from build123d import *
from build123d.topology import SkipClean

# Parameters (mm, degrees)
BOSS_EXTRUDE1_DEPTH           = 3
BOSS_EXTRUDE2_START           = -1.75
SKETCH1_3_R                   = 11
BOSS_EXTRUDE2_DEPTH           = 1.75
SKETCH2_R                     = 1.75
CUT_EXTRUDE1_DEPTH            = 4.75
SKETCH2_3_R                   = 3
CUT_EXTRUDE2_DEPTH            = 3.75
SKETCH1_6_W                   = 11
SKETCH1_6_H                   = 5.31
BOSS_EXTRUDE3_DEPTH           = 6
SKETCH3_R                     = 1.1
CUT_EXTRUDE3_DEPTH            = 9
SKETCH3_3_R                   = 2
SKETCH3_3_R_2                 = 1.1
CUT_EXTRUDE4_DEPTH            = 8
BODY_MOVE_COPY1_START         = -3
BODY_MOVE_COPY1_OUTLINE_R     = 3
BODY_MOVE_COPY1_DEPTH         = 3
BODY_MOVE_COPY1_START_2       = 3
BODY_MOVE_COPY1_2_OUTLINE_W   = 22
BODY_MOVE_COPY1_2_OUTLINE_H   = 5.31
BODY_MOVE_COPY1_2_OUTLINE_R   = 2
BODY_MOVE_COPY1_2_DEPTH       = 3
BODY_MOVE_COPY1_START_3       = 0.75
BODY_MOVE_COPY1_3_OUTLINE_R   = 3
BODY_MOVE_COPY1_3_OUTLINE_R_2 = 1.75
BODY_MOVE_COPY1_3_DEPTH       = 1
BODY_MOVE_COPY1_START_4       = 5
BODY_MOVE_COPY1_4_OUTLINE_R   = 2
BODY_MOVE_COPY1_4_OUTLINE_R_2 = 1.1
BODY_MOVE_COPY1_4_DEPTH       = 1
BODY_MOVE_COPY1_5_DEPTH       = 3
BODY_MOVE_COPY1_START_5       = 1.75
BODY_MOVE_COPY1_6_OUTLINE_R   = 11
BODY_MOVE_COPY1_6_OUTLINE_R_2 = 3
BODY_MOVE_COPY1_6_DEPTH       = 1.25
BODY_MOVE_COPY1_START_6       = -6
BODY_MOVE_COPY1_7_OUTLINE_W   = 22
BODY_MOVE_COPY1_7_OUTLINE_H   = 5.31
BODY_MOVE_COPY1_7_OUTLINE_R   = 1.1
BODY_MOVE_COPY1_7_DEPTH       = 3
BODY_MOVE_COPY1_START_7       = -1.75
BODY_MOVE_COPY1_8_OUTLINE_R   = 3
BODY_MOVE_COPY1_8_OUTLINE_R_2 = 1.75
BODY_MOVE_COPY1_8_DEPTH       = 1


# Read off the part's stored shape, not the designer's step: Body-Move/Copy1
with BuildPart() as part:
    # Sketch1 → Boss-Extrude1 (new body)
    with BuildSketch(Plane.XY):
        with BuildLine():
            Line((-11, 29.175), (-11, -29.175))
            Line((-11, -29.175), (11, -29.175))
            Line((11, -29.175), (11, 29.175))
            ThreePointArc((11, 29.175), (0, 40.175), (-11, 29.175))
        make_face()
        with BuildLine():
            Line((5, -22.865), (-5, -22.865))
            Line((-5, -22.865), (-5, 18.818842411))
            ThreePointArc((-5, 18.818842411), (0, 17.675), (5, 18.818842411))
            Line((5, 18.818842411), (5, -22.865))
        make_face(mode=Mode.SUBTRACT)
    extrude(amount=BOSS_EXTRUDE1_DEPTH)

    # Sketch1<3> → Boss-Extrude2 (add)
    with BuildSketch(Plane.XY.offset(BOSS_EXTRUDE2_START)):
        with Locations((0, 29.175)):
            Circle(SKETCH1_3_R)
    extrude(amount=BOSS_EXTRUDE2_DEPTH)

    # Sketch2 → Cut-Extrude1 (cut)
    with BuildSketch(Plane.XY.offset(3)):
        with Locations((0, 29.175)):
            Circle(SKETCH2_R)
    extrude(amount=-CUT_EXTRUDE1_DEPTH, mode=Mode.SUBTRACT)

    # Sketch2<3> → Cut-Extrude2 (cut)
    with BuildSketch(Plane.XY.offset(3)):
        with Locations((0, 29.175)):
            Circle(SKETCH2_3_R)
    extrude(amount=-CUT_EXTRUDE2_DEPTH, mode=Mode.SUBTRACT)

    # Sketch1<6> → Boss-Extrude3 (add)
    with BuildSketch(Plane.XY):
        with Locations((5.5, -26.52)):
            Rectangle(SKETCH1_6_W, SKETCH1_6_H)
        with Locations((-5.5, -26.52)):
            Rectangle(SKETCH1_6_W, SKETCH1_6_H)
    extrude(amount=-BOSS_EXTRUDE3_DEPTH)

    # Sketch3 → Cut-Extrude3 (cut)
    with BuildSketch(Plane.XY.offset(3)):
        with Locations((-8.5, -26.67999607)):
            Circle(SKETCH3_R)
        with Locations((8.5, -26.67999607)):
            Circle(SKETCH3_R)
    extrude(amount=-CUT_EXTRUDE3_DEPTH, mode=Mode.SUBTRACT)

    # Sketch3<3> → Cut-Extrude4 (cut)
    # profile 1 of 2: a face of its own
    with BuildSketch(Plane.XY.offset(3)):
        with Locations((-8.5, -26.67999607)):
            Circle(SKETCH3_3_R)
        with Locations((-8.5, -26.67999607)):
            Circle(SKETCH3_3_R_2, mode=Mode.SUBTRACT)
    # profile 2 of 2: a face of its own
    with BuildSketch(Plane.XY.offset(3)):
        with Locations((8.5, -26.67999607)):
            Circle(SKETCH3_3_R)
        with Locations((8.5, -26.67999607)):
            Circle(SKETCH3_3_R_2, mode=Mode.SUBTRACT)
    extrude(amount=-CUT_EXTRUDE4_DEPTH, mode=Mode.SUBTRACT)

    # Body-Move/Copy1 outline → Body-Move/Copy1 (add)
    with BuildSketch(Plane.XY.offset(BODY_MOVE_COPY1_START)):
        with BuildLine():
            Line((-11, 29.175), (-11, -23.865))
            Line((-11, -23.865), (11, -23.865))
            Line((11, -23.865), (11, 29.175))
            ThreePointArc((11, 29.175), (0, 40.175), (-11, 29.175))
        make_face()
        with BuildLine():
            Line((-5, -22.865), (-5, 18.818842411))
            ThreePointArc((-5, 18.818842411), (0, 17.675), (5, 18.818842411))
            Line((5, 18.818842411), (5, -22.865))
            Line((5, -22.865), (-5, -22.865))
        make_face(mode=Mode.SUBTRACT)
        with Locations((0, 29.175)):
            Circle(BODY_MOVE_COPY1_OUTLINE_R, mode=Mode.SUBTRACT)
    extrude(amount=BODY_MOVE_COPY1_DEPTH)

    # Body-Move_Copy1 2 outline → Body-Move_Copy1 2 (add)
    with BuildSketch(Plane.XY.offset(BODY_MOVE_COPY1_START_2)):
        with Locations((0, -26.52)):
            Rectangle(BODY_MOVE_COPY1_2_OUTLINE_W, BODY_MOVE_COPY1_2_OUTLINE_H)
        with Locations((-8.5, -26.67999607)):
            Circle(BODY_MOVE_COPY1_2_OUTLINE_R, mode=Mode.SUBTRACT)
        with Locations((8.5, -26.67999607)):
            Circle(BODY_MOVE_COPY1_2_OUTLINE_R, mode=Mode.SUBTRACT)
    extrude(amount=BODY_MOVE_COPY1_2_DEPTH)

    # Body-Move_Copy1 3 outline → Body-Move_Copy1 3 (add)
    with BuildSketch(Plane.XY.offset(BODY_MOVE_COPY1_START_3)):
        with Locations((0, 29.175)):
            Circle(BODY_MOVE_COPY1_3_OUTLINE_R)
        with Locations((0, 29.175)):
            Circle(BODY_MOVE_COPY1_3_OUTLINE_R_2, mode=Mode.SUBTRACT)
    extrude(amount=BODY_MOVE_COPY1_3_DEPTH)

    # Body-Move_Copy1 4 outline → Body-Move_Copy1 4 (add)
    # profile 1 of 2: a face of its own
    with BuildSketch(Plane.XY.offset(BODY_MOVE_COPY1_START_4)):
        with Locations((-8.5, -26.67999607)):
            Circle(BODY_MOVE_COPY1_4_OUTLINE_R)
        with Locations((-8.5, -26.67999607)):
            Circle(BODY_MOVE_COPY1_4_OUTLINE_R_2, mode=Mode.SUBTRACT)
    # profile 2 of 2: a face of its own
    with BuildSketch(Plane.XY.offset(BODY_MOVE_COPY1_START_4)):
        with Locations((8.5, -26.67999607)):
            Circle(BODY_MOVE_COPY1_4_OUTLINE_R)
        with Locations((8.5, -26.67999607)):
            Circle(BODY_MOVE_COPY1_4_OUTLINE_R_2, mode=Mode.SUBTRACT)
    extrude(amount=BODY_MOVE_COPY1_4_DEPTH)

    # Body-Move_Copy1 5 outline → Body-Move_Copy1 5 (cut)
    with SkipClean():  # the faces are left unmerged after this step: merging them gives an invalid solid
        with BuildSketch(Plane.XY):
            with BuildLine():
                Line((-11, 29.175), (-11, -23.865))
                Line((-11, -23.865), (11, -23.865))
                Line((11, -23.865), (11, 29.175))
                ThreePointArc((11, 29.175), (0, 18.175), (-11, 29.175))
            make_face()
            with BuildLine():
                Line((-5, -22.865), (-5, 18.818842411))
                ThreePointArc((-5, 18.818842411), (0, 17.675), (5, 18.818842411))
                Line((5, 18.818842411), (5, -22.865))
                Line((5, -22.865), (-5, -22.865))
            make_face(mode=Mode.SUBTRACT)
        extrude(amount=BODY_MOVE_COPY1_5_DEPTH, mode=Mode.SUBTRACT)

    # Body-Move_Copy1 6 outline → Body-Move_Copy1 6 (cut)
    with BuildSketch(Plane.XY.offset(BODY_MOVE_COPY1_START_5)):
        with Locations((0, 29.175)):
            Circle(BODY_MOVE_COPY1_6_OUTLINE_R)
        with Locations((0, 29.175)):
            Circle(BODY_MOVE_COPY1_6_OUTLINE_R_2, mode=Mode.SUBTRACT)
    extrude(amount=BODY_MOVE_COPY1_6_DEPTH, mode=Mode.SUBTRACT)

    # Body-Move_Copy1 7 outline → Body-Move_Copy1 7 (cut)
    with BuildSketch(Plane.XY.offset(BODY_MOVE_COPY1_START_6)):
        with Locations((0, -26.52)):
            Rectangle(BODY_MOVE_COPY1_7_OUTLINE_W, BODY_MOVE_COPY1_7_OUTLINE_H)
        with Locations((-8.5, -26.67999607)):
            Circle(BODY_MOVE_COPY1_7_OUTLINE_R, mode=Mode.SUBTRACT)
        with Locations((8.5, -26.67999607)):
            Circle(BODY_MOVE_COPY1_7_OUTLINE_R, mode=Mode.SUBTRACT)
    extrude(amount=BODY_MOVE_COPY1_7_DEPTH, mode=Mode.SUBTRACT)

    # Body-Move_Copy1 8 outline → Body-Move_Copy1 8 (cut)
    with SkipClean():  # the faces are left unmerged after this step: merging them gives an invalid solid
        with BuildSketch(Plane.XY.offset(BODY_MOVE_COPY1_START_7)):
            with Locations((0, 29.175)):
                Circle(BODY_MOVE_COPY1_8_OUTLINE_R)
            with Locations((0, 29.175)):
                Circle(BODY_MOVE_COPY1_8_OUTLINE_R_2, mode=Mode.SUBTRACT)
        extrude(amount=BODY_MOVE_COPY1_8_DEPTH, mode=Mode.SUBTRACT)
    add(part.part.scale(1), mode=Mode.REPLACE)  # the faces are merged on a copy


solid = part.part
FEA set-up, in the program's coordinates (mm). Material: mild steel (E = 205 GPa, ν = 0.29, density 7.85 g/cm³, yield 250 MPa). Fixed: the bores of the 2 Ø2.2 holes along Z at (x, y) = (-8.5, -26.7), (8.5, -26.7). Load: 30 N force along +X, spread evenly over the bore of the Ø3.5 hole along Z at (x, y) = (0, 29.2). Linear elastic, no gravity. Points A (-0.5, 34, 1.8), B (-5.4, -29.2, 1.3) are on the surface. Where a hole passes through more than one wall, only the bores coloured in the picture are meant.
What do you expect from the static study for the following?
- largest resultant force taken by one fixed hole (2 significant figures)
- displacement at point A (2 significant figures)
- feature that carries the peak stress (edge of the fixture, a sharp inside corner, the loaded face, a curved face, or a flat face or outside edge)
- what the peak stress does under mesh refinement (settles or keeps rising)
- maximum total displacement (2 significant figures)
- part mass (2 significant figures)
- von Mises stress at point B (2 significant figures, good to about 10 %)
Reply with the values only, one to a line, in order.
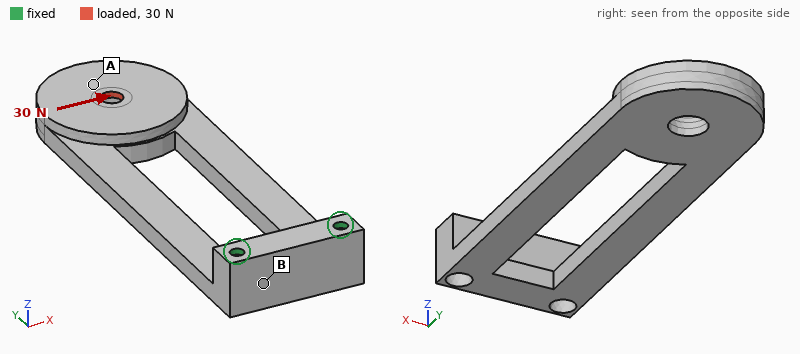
88 N
34 µm
edge of the fixture
keeps rising
36 µm
33 g
11 MPa
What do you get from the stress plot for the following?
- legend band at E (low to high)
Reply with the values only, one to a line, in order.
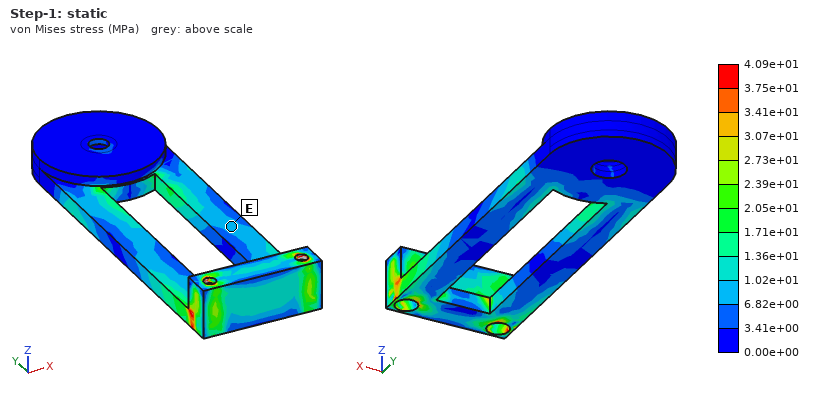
6.82e+00 to 1.02e+01 MPa
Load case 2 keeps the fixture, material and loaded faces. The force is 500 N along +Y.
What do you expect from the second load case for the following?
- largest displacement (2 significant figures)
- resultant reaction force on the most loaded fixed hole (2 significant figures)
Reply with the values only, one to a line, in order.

0.36 mm
250 N
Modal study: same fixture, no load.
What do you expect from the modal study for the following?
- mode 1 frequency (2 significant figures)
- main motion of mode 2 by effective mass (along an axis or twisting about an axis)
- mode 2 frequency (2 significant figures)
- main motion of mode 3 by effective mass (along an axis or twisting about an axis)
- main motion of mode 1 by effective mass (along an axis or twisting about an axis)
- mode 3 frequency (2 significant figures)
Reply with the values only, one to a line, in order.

340 Hz
along X
1200 Hz
twisting about Y
along Z
2300 Hz
